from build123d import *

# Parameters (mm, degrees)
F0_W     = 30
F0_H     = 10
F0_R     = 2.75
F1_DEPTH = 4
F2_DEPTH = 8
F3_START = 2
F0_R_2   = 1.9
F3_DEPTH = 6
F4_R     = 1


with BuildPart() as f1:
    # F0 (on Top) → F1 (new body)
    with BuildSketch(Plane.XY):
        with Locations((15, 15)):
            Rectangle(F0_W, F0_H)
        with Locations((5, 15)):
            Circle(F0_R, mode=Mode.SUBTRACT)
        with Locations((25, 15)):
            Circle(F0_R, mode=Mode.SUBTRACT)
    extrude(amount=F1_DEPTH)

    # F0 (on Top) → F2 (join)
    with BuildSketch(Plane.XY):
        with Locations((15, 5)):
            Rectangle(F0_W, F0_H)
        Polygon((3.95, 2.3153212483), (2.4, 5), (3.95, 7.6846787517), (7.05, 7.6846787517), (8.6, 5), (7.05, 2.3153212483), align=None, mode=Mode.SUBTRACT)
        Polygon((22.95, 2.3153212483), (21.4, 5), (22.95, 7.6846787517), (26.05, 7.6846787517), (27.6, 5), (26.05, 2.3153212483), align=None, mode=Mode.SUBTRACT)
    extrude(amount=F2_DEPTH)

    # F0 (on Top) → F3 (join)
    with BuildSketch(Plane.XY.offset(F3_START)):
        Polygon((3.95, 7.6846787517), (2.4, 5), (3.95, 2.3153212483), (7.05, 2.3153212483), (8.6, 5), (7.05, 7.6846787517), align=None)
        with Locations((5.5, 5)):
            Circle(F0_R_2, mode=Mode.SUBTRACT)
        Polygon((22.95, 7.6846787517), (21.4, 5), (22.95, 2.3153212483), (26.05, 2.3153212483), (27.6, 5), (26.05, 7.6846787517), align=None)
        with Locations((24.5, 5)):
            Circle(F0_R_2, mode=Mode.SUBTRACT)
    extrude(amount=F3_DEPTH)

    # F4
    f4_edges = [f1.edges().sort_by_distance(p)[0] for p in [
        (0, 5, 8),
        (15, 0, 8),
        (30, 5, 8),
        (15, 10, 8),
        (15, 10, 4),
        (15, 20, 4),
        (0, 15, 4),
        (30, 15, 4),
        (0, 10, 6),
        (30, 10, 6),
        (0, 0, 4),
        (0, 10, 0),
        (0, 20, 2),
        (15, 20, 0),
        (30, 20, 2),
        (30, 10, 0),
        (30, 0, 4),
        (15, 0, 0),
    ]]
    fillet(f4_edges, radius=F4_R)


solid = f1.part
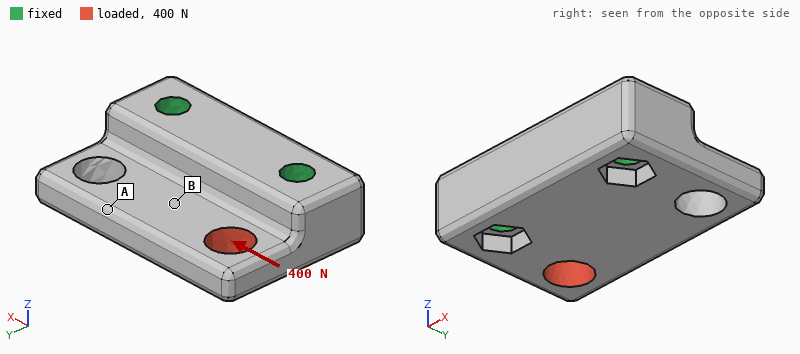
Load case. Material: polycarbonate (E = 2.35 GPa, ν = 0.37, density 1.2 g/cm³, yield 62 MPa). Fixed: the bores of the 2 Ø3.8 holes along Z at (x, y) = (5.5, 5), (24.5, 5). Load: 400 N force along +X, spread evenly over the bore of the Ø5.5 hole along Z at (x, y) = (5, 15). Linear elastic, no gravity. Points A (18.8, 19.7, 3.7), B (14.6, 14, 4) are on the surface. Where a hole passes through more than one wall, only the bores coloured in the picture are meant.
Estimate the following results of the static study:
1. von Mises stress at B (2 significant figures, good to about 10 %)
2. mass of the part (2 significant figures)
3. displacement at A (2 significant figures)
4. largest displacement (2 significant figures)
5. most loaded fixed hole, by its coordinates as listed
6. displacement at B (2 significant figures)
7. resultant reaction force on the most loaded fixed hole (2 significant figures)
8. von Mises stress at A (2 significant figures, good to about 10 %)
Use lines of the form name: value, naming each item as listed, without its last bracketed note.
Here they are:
von Mises stress at B: 7.2 MPa
mass of the part: 3.8 g
displacement at A: 0.058 mm
largest displacement: 0.13 mm
most loaded fixed hole, by its coordinates as listed: (5.5, 5)
displacement at B: 0.041 mm
resultant reaction force on the most loaded fixed hole: 290 N
von Mises stress at A: 3.2 MPa
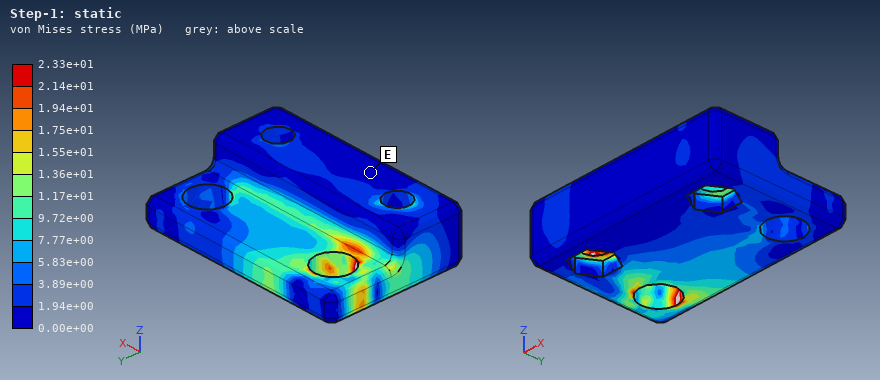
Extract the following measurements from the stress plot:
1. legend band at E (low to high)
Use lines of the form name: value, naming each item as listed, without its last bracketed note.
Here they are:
legend band at E: 0.00e+00 to 1.94e+00 MPa
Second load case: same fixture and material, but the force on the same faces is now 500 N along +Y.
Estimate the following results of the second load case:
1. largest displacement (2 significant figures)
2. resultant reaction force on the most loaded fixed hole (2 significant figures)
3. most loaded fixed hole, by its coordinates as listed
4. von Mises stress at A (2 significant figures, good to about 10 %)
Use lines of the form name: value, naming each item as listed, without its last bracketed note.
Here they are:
largest displacement: 0.17 mm
resultant reaction force on the most loaded fixed hole: 490 N
most loaded fixed hole, by its coordinates as listed: (5.5, 5)
von Mises stress at A: 2.2 MPa
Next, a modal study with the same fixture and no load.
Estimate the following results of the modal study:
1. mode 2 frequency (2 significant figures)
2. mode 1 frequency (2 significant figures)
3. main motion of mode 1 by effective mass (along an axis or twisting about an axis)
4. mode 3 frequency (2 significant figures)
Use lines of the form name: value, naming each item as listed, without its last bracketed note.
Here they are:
mode 2 frequency: 7200 Hz
mode 1 frequency: 5100 Hz
main motion of mode 1 by effective mass: along Z
mode 3 frequency: 10 kHz
